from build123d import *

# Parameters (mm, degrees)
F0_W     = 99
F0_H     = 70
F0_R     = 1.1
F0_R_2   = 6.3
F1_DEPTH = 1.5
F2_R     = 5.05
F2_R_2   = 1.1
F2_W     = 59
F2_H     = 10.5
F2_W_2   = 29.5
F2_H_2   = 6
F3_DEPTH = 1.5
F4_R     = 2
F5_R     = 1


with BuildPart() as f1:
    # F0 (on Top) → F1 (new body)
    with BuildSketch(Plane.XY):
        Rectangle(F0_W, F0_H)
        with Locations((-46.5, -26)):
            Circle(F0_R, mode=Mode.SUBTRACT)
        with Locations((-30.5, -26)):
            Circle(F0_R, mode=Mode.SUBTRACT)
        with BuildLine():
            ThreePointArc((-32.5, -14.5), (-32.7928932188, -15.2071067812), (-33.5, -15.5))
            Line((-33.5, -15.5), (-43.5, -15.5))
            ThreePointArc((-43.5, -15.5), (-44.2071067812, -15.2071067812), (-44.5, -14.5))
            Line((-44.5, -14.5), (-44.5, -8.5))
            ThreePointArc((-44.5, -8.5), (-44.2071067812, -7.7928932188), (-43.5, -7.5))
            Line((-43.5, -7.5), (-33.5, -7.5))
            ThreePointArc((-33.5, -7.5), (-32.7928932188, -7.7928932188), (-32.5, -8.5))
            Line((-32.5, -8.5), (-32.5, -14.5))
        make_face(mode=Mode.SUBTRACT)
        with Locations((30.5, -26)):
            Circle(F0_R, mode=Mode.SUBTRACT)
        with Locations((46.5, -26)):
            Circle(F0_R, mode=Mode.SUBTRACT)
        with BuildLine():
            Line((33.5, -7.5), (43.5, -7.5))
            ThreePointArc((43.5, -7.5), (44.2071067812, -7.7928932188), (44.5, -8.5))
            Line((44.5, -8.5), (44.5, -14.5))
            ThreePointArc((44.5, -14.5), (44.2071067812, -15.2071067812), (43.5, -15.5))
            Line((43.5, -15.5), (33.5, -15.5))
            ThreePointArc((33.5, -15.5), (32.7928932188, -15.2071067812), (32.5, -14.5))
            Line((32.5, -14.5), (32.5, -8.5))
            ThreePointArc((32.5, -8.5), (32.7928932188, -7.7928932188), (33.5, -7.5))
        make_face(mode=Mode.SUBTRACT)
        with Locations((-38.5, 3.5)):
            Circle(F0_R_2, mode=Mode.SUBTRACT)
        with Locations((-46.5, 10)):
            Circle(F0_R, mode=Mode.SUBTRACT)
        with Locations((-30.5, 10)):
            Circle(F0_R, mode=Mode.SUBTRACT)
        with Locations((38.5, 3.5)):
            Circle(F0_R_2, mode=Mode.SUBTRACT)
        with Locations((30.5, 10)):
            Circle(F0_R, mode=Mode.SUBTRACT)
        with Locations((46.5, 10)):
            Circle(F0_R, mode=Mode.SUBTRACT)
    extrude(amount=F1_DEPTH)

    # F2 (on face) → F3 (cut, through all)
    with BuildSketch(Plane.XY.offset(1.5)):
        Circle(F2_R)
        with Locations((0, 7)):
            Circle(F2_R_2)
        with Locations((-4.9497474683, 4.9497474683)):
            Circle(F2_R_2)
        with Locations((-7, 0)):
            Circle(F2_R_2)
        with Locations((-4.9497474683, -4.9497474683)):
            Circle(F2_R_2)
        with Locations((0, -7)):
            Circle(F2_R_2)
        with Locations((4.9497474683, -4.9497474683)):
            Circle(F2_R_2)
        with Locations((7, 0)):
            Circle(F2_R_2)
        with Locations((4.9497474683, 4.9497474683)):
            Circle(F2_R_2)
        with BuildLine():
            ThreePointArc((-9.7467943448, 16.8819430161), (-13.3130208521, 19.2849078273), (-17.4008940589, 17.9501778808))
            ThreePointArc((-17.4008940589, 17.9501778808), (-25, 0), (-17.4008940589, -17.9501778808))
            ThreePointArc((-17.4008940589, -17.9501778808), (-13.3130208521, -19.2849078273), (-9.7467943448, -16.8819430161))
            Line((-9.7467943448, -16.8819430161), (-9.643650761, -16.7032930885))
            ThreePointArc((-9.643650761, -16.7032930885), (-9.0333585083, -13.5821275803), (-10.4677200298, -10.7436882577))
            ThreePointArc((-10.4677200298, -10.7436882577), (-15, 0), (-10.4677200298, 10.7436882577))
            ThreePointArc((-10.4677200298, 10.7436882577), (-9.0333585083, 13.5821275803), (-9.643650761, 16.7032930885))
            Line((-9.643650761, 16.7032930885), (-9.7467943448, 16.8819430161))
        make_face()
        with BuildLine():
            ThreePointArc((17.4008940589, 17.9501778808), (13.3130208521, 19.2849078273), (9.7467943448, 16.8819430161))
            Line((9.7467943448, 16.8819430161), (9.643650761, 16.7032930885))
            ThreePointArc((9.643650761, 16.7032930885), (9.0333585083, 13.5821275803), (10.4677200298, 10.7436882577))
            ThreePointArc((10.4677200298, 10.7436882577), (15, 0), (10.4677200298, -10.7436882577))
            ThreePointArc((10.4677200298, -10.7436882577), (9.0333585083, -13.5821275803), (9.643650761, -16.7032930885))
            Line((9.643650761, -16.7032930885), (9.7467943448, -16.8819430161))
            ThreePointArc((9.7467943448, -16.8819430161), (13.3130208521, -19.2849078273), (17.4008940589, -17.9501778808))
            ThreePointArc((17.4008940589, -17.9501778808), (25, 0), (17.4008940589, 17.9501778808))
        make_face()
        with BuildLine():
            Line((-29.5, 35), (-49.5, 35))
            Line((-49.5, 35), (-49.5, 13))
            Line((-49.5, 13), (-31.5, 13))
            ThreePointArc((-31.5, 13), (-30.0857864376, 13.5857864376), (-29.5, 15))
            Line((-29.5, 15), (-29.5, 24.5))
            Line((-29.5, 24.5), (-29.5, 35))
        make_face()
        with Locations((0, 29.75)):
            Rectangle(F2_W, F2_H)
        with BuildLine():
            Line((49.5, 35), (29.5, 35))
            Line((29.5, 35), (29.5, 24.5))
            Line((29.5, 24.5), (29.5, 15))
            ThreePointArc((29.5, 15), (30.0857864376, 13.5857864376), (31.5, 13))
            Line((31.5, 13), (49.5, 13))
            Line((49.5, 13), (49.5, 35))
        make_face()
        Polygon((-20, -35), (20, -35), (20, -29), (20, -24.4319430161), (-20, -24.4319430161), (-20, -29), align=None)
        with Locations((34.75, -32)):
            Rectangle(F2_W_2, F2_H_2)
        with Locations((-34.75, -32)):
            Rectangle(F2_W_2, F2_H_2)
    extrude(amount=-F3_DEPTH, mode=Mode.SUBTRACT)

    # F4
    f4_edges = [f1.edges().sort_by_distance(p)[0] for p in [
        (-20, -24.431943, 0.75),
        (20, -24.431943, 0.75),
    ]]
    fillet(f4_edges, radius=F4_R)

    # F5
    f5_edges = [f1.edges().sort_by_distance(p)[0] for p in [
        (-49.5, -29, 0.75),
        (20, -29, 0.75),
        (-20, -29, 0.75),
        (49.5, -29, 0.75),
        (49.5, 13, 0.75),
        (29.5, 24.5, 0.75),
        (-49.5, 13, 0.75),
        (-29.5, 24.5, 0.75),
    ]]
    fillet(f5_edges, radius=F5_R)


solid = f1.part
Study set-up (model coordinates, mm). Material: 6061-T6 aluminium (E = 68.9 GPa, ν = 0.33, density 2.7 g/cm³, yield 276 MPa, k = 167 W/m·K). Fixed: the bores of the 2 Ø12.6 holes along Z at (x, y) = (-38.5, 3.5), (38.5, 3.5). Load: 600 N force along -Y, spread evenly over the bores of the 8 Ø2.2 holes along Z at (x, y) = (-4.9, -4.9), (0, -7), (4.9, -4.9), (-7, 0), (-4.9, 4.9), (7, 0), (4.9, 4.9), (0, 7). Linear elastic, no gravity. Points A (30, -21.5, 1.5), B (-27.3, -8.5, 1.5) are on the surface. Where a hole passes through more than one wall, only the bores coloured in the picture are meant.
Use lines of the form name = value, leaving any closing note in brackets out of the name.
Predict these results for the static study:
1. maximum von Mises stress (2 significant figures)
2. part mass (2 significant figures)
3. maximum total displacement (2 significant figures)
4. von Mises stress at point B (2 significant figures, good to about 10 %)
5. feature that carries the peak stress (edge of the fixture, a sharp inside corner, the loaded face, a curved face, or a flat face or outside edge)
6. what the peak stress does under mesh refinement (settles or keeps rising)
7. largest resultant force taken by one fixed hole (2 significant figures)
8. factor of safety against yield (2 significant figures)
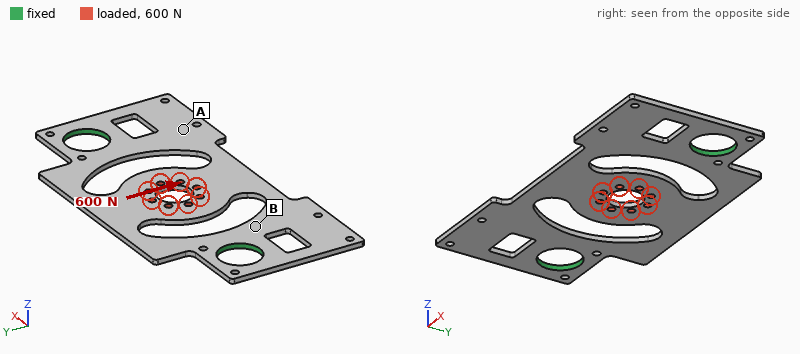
maximum von Mises stress = 98 MPa
part mass = 13 g
maximum total displacement = 43 µm
von Mises stress at point B = 19 MPa
feature that carries the peak stress = a curved face
what the peak stress does under mesh refinement = settles
largest resultant force taken by one fixed hole = 300 N
factor of safety against yield = 2.8
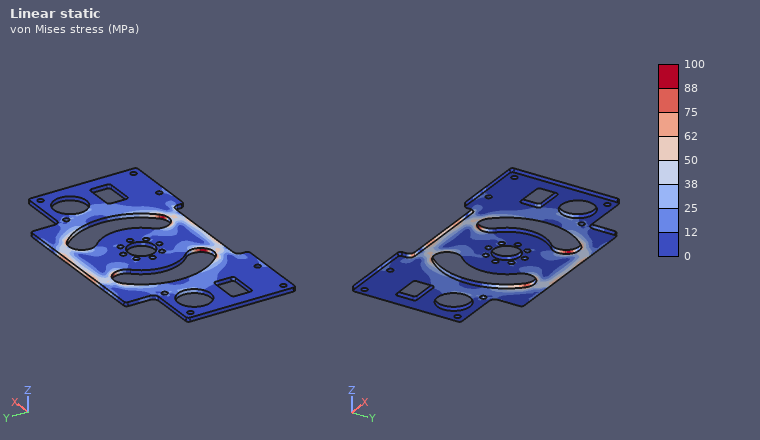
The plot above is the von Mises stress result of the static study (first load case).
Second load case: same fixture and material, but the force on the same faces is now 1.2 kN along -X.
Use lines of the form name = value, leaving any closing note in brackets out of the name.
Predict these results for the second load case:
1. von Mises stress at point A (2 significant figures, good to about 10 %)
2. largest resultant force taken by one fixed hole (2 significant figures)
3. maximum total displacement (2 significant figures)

von Mises stress at point A = 16 MPa
largest resultant force taken by one fixed hole = 600 N
maximum total displacement = 74 µm
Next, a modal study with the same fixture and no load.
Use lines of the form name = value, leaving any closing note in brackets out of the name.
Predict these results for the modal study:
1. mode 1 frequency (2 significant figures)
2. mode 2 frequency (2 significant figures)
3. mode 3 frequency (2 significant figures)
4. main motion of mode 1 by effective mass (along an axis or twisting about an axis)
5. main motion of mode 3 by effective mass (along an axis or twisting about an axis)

mode 1 frequency = 890 Hz
mode 2 frequency = 1100 Hz
mode 3 frequency = 1400 Hz
main motion of mode 1 by effective mass = along Z
main motion of mode 3 by effective mass = twisting about Y
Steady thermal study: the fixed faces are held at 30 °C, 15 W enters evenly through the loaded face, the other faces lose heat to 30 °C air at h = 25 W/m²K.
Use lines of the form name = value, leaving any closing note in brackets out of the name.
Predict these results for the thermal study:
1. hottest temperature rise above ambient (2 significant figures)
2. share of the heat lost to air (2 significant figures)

hottest temperature rise above ambient = 69 K
share of the heat lost to air = 31 %
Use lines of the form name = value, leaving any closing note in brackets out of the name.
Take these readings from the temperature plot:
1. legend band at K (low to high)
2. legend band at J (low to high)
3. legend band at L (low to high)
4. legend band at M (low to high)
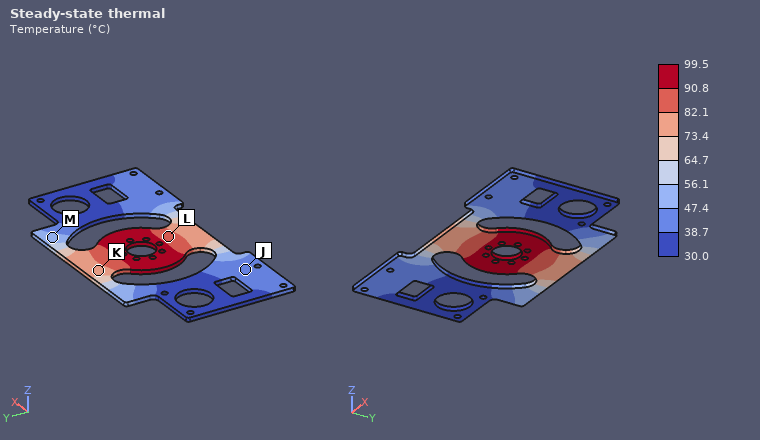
legend band at K = 73.4 to 82.1 °C
legend band at J = 38.7 to 47.4 °C
legend band at L = 82.1 to 90.8 °C
legend band at M = 47.4 to 56.1 °C
